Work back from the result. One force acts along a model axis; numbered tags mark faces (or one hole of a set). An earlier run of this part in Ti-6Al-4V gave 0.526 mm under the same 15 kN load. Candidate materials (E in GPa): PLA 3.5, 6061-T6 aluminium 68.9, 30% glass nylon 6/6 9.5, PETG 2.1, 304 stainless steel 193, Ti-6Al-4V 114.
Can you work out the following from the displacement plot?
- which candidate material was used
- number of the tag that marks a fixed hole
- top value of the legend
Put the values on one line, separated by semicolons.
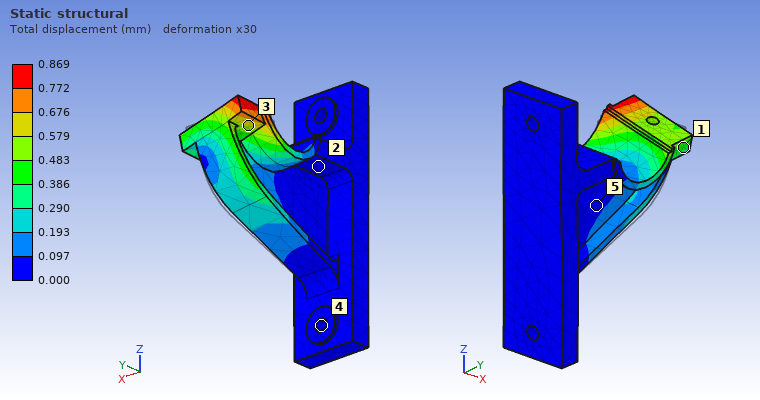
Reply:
6061-T6 aluminium; 4; 0.869 mm
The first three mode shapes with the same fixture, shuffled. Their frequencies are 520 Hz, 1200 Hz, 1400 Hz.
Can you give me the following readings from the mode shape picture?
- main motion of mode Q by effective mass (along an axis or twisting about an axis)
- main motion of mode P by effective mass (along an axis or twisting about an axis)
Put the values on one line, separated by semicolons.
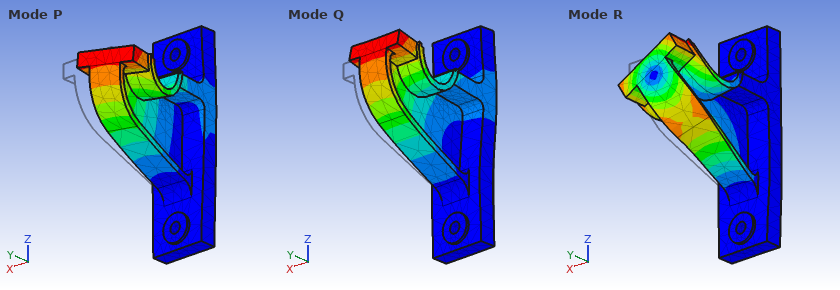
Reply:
along Z; along X
